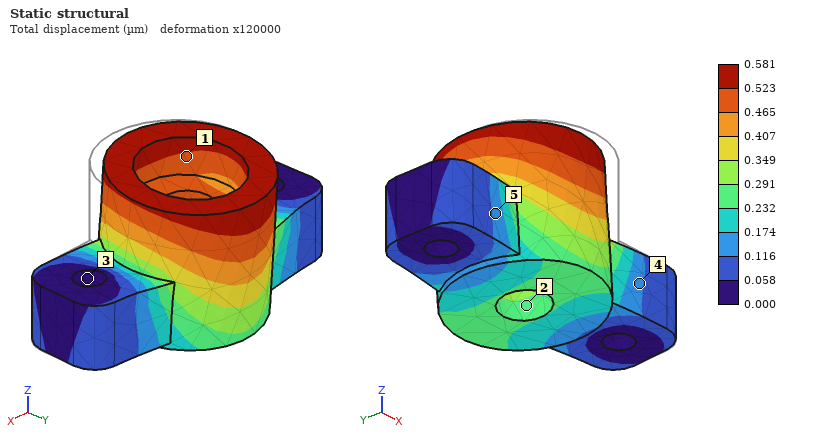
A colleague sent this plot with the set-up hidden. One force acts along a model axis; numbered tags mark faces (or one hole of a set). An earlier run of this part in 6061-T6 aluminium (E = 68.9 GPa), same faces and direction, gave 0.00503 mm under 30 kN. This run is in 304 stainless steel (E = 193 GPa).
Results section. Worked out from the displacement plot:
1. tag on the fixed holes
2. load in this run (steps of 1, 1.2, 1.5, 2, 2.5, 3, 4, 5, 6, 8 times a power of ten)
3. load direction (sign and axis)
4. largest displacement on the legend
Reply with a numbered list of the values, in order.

1. 3
2. 10 kN
3. +Y
4. 0.581 µm
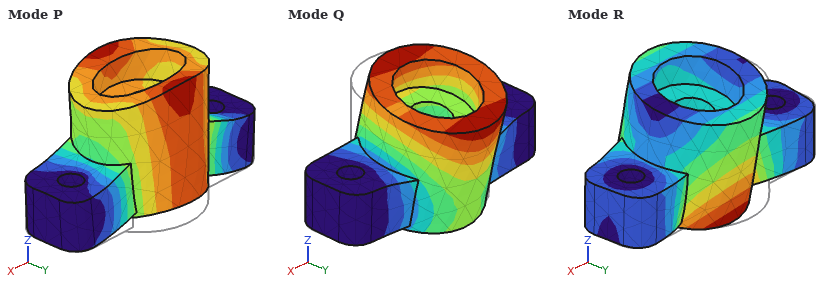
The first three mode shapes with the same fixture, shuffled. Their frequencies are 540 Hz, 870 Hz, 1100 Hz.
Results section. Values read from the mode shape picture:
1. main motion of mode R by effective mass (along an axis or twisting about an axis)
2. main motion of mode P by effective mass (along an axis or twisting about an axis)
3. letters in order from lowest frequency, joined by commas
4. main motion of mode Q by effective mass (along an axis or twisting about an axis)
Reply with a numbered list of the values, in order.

1. along Y
2. along Z
3. Q, P, R
4. along Y
